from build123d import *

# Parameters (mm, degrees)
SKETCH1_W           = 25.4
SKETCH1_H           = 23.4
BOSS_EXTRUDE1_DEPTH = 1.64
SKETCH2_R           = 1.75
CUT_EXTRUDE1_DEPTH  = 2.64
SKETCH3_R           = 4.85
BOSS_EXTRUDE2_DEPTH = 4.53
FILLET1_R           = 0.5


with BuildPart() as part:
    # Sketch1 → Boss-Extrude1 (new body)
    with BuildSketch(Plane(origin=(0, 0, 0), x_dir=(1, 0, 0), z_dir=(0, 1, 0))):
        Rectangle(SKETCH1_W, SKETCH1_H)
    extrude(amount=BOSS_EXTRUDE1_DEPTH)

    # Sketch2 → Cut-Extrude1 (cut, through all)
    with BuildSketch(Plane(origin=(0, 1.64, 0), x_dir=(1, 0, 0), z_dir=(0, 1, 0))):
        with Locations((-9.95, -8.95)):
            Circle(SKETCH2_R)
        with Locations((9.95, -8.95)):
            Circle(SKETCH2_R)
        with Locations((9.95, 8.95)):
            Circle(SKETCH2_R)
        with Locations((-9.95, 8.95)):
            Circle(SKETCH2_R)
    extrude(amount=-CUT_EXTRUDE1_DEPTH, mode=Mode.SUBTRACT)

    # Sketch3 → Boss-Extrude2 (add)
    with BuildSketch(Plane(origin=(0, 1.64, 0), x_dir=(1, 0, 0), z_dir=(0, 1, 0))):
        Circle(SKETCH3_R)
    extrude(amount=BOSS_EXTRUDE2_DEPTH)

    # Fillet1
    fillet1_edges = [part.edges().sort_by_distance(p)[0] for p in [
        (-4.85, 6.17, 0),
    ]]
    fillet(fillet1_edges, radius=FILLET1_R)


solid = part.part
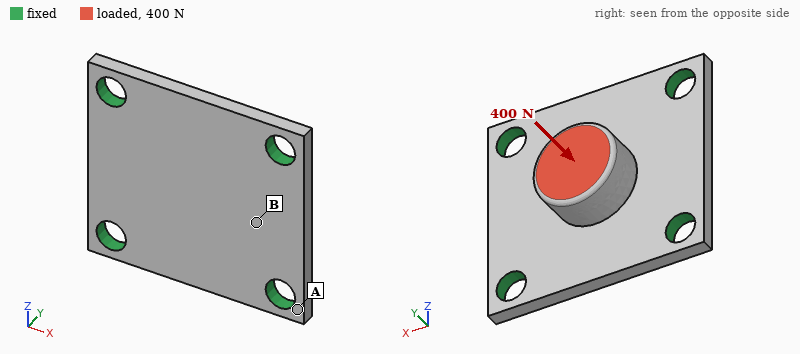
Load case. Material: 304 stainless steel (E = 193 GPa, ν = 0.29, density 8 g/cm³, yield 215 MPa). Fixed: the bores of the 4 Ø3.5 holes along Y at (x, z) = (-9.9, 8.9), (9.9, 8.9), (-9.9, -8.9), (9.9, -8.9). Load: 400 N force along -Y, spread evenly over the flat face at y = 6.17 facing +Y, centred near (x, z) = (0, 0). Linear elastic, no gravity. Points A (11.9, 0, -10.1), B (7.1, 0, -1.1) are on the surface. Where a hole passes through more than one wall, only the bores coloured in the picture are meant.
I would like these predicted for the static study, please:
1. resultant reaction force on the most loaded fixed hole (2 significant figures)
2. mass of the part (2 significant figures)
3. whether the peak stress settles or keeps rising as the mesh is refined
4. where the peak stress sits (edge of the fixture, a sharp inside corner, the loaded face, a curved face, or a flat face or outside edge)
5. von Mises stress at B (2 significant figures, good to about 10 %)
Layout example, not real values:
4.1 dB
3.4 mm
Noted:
100 N
10.0 g
keeps rising
edge of the fixture
34 MPa
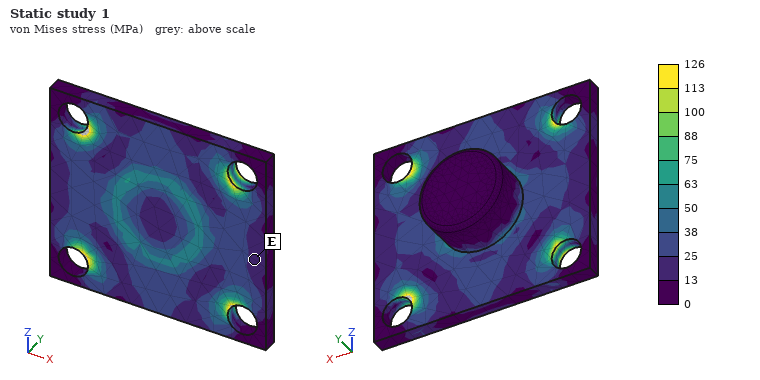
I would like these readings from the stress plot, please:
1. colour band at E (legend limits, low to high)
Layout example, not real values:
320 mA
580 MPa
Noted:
13 to 25 MPa
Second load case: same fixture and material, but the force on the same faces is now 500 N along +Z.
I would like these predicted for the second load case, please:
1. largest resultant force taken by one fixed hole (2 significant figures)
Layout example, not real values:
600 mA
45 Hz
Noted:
170 N
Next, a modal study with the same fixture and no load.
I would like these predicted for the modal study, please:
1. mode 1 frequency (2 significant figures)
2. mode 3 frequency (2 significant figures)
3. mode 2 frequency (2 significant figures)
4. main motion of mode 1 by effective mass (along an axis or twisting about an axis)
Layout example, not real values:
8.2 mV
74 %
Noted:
16 kHz
27 kHz
24 kHz
along Y
